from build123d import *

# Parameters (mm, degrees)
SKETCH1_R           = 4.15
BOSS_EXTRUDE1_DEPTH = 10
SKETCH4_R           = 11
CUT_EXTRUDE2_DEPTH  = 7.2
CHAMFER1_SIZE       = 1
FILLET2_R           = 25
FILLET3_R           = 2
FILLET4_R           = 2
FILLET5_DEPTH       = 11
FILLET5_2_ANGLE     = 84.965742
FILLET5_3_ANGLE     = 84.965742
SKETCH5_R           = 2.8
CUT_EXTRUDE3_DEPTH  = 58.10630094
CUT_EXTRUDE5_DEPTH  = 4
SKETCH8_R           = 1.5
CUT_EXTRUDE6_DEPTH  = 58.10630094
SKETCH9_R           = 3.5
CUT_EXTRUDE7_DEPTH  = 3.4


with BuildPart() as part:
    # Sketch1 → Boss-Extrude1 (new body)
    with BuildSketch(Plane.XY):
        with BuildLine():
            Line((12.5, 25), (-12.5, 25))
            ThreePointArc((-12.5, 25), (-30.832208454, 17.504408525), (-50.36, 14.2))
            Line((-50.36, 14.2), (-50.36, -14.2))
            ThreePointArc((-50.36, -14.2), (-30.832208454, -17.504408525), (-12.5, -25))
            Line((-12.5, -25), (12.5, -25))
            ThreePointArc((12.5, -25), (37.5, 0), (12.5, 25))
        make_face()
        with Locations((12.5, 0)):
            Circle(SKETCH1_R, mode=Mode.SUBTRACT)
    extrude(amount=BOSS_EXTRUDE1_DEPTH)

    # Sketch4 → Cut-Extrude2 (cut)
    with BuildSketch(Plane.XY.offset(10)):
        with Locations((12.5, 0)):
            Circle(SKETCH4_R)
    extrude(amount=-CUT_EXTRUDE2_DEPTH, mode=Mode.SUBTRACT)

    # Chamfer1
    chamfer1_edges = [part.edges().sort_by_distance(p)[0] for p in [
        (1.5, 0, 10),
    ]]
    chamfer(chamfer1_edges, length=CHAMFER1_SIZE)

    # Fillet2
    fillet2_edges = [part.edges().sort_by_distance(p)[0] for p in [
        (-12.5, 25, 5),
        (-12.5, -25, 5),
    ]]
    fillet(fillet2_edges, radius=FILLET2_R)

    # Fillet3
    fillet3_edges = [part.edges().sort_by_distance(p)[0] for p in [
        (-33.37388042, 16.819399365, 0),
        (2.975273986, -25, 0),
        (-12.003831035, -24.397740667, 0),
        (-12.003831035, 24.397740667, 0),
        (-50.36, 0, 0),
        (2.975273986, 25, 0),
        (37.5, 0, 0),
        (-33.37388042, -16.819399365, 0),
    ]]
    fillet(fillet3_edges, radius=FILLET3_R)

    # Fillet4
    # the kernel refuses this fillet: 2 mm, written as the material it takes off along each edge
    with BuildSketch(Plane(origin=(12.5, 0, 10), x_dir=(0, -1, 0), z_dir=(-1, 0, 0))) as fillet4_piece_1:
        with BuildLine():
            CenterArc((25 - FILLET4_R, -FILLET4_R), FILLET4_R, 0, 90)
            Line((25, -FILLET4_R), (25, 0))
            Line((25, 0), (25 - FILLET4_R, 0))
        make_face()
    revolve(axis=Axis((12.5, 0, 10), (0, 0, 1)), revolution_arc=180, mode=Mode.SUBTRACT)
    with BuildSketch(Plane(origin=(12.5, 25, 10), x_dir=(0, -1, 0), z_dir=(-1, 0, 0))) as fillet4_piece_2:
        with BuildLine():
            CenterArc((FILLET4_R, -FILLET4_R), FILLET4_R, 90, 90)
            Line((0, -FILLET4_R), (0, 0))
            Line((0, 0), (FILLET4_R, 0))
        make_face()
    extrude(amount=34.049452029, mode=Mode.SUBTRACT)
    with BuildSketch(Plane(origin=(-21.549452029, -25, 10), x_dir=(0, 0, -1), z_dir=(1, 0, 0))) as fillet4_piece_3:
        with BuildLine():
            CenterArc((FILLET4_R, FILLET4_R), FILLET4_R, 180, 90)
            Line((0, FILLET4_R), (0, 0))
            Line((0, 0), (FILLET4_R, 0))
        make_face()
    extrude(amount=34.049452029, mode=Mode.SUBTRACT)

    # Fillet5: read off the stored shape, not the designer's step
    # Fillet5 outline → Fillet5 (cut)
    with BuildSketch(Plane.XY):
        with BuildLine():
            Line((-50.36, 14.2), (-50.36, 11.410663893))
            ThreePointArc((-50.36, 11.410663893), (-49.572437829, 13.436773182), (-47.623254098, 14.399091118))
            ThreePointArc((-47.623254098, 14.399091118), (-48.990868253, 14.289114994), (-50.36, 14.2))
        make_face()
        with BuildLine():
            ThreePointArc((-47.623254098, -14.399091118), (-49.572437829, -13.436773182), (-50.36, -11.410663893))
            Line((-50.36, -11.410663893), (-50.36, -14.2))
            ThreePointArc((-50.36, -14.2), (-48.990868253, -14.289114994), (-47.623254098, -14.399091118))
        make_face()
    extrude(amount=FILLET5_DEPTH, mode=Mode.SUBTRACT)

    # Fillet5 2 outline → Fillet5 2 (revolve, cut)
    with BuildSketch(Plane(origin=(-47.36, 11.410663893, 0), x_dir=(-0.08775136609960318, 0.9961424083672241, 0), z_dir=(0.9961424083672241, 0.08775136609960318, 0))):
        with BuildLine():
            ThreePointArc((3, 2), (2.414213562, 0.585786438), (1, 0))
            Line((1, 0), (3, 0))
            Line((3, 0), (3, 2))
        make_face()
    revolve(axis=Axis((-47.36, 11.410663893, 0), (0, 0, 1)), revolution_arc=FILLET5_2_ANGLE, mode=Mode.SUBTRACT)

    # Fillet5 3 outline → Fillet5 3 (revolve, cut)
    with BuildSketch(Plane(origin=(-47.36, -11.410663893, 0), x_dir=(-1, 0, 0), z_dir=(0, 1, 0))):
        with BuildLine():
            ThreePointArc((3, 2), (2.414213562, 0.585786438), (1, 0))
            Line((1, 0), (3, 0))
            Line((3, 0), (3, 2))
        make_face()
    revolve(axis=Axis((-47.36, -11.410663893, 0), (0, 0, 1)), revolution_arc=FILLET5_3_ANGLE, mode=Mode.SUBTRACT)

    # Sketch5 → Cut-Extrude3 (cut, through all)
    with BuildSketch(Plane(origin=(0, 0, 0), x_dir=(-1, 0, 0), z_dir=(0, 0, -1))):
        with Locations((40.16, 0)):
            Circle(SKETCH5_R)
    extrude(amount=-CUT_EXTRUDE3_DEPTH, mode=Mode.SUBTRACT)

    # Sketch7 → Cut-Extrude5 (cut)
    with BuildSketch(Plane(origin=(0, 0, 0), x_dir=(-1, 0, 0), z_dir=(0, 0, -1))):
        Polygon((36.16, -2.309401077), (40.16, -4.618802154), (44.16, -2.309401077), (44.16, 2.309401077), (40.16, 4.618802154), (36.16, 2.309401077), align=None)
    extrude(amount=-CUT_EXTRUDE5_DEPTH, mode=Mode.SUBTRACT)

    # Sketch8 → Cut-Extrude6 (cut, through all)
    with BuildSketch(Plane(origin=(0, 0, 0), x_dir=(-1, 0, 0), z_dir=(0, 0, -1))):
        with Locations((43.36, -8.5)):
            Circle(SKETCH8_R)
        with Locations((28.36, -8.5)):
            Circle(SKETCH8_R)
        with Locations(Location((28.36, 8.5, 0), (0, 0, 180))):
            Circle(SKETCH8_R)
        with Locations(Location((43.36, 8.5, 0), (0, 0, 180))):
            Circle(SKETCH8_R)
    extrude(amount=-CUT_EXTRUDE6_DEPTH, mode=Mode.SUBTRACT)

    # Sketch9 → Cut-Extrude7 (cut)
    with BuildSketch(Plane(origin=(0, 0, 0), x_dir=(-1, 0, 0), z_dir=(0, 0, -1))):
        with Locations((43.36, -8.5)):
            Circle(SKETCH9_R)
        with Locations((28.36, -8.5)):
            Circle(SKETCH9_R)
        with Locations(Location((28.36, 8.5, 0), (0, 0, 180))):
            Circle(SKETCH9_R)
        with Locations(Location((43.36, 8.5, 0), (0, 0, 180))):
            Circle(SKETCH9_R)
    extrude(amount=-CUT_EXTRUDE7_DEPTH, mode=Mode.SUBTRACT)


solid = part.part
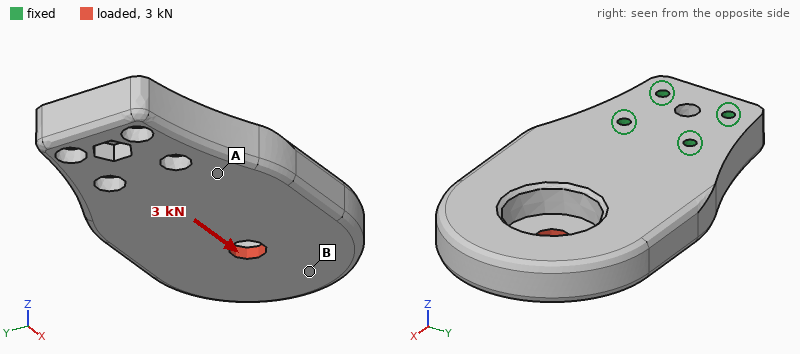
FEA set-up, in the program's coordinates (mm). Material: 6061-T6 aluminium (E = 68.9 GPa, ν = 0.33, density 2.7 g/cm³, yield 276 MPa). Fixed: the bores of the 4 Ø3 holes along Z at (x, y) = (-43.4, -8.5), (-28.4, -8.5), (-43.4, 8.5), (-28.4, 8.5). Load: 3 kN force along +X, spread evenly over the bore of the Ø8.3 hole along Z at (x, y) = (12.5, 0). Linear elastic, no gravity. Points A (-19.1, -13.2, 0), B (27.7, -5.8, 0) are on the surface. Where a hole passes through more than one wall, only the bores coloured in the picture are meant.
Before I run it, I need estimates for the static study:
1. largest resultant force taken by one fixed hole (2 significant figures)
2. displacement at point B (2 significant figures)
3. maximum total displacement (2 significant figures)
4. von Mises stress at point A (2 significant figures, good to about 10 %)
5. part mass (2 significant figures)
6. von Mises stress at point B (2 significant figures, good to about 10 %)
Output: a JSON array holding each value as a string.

["1.0 kN", "0.087 mm", "0.11 mm", "22 MPa", "85 g", "9.6 MPa"]
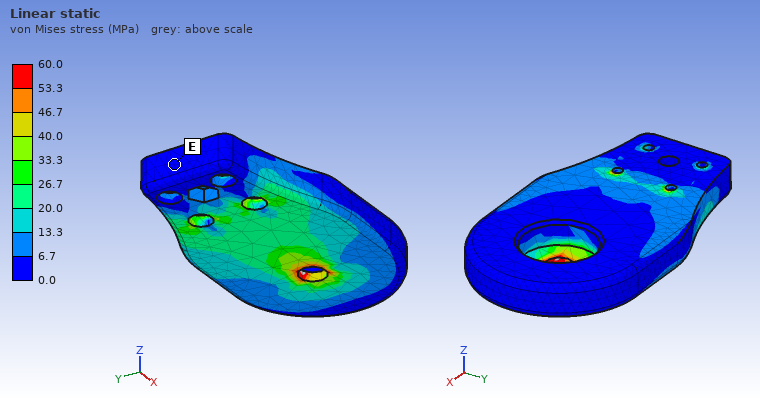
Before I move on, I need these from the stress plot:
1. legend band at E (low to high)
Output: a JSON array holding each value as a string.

["0.0 to 6.7 MPa"]
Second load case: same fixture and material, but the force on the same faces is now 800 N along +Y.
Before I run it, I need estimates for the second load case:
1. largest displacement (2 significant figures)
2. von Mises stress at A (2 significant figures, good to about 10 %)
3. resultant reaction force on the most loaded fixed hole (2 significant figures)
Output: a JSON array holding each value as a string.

["23 µm", "7.0 MPa", "1.2 kN"]
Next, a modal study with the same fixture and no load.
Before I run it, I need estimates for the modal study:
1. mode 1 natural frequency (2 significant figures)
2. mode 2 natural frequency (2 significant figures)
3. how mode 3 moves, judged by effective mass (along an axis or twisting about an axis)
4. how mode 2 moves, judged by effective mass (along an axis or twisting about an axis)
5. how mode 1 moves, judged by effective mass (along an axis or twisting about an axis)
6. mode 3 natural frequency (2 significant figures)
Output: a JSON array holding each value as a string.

["1800 Hz", "4700 Hz", "along Y", "along Y", "along Z", "5000 Hz"]
